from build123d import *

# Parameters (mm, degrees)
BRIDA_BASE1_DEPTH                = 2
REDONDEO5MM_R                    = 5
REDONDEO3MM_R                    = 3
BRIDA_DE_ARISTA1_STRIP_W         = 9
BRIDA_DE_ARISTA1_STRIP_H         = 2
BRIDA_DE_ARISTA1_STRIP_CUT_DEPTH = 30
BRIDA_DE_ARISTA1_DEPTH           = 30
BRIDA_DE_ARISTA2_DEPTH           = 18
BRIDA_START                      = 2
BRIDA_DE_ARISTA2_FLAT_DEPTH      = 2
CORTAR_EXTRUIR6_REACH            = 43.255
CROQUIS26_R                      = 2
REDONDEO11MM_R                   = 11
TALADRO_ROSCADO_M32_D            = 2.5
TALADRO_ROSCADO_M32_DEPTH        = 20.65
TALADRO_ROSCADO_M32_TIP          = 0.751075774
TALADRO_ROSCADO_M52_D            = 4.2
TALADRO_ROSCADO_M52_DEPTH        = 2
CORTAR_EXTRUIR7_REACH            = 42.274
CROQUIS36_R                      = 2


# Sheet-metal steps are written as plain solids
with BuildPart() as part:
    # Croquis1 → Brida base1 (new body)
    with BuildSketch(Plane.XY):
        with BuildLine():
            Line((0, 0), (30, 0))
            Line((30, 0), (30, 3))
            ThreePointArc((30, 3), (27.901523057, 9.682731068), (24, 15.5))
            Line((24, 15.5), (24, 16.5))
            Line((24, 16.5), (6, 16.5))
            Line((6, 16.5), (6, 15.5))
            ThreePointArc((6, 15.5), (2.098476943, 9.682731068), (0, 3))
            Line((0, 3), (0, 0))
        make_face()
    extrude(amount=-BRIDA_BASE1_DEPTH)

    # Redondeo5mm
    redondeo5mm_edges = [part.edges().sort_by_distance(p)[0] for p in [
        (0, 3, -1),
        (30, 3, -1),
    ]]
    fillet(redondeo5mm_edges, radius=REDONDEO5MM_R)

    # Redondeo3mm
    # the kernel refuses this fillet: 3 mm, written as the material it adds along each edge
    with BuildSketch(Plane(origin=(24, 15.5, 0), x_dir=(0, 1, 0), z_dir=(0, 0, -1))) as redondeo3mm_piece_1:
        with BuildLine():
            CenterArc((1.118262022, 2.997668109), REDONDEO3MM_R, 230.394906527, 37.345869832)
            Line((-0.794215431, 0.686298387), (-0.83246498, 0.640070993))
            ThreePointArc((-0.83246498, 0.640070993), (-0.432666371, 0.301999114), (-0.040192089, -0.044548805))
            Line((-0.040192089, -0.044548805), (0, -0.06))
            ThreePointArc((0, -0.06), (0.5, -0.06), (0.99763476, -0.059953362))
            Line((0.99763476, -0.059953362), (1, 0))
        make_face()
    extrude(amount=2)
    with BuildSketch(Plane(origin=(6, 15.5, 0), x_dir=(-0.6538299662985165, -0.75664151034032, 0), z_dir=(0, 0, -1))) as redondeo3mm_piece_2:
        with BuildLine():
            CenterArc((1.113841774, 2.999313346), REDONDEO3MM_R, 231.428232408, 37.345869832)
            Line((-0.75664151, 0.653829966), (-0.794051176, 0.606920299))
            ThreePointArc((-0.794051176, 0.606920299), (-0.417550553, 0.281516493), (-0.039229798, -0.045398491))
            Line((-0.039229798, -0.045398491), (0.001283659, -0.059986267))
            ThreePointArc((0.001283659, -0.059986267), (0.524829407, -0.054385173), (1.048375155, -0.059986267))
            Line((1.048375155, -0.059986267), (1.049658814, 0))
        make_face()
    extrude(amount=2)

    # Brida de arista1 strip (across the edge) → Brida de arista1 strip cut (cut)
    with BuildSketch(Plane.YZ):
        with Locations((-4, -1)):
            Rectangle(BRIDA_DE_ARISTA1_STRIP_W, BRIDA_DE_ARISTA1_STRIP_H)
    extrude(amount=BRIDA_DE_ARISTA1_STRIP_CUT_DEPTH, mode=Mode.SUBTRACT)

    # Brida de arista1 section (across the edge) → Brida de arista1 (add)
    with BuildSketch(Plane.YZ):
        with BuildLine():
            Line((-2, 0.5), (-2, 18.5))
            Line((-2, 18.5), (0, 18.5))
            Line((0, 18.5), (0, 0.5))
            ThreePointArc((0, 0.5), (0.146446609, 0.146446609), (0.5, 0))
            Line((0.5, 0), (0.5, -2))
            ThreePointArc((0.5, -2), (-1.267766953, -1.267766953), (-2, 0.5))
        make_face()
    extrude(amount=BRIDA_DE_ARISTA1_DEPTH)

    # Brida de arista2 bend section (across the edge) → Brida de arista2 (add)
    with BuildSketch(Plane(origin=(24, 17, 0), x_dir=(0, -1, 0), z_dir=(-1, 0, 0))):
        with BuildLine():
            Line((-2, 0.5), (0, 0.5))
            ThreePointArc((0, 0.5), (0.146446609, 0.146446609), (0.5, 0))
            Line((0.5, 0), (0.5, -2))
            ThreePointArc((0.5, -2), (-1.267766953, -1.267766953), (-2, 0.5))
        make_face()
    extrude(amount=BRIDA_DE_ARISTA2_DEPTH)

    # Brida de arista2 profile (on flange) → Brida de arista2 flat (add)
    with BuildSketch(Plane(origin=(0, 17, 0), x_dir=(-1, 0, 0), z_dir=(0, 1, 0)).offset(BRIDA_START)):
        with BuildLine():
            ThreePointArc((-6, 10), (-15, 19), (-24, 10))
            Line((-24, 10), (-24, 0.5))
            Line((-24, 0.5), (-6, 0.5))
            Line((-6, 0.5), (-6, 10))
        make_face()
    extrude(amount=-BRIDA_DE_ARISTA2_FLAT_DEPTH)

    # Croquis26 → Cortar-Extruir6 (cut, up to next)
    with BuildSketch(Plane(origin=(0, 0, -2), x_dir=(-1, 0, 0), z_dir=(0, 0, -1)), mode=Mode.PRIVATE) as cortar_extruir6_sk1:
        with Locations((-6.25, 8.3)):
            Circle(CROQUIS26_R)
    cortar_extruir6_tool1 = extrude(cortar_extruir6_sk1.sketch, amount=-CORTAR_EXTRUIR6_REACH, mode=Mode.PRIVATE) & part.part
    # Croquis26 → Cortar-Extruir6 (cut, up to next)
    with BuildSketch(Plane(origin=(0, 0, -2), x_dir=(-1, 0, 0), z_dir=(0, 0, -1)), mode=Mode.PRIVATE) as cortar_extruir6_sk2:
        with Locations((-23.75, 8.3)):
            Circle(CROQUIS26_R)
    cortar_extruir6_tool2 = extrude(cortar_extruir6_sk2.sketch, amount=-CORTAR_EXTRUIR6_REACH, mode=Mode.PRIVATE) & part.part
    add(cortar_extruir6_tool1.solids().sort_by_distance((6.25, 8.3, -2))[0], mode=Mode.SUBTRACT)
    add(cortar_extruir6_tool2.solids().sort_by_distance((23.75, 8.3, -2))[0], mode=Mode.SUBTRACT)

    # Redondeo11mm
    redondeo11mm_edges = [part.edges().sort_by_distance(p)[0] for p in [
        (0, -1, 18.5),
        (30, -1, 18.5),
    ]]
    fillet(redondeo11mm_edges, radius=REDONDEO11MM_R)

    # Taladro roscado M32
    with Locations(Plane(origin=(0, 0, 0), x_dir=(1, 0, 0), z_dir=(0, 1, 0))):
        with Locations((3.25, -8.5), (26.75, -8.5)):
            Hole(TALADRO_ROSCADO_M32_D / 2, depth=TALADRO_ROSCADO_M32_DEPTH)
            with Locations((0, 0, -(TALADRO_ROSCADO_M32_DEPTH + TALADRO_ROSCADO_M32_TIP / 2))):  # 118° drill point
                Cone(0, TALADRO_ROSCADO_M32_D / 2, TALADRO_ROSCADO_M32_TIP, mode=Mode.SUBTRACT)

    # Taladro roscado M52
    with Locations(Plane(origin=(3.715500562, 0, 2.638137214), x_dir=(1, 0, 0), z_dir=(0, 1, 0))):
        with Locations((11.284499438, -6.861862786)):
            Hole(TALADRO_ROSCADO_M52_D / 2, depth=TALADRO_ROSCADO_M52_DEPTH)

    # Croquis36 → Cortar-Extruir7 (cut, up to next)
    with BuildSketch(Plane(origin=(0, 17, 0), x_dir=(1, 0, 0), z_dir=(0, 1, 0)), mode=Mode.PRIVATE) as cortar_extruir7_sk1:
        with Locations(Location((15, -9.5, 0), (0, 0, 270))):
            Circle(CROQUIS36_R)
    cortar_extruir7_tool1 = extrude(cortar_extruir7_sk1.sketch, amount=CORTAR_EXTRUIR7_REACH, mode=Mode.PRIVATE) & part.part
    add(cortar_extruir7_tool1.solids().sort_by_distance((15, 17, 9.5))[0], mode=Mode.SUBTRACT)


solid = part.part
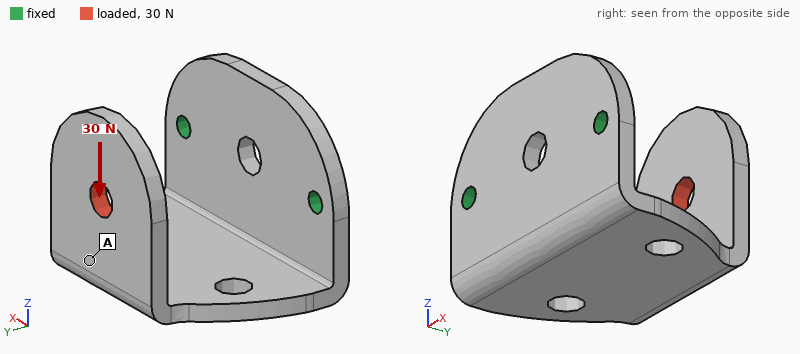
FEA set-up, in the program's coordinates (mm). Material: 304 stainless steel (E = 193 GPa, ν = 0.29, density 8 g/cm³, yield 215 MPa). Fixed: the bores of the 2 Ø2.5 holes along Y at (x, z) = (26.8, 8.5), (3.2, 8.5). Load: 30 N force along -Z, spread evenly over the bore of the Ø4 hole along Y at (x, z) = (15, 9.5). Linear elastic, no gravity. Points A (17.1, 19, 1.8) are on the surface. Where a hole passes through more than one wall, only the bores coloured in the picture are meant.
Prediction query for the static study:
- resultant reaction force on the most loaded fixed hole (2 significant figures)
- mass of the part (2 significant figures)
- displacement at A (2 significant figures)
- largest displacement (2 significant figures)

16 N
20 g
50 µm
73 µm
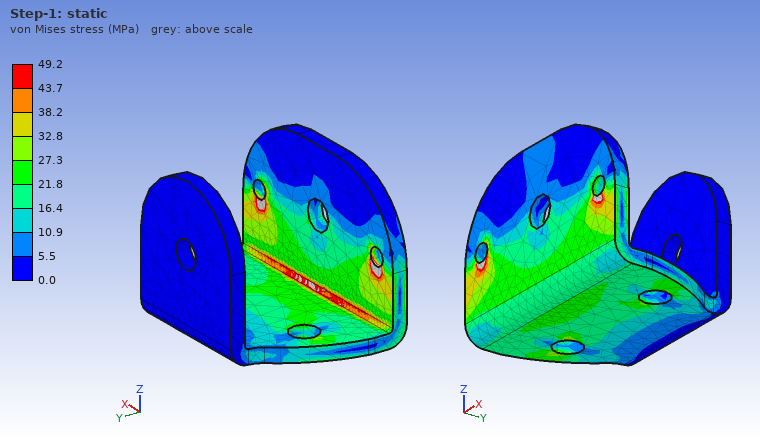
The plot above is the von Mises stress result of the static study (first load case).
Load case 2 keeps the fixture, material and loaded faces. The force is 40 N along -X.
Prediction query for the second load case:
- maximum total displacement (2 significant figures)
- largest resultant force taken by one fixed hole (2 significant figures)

41 µm
38 N
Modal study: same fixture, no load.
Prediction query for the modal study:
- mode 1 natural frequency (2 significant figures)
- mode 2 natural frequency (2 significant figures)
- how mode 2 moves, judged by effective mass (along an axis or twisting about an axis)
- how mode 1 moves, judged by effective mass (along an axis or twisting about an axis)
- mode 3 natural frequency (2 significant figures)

1400 Hz
2600 Hz
along X
along Z
3200 Hz
